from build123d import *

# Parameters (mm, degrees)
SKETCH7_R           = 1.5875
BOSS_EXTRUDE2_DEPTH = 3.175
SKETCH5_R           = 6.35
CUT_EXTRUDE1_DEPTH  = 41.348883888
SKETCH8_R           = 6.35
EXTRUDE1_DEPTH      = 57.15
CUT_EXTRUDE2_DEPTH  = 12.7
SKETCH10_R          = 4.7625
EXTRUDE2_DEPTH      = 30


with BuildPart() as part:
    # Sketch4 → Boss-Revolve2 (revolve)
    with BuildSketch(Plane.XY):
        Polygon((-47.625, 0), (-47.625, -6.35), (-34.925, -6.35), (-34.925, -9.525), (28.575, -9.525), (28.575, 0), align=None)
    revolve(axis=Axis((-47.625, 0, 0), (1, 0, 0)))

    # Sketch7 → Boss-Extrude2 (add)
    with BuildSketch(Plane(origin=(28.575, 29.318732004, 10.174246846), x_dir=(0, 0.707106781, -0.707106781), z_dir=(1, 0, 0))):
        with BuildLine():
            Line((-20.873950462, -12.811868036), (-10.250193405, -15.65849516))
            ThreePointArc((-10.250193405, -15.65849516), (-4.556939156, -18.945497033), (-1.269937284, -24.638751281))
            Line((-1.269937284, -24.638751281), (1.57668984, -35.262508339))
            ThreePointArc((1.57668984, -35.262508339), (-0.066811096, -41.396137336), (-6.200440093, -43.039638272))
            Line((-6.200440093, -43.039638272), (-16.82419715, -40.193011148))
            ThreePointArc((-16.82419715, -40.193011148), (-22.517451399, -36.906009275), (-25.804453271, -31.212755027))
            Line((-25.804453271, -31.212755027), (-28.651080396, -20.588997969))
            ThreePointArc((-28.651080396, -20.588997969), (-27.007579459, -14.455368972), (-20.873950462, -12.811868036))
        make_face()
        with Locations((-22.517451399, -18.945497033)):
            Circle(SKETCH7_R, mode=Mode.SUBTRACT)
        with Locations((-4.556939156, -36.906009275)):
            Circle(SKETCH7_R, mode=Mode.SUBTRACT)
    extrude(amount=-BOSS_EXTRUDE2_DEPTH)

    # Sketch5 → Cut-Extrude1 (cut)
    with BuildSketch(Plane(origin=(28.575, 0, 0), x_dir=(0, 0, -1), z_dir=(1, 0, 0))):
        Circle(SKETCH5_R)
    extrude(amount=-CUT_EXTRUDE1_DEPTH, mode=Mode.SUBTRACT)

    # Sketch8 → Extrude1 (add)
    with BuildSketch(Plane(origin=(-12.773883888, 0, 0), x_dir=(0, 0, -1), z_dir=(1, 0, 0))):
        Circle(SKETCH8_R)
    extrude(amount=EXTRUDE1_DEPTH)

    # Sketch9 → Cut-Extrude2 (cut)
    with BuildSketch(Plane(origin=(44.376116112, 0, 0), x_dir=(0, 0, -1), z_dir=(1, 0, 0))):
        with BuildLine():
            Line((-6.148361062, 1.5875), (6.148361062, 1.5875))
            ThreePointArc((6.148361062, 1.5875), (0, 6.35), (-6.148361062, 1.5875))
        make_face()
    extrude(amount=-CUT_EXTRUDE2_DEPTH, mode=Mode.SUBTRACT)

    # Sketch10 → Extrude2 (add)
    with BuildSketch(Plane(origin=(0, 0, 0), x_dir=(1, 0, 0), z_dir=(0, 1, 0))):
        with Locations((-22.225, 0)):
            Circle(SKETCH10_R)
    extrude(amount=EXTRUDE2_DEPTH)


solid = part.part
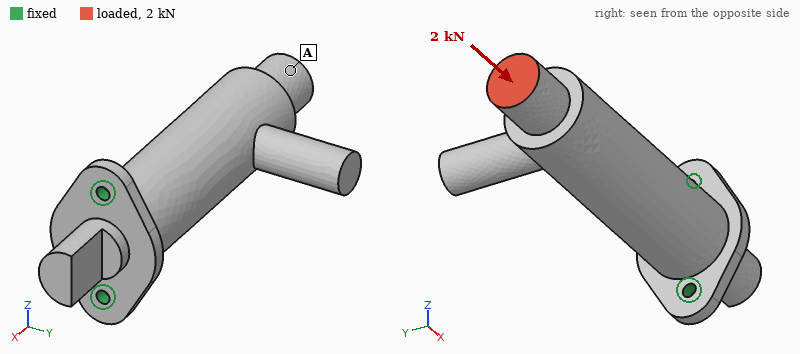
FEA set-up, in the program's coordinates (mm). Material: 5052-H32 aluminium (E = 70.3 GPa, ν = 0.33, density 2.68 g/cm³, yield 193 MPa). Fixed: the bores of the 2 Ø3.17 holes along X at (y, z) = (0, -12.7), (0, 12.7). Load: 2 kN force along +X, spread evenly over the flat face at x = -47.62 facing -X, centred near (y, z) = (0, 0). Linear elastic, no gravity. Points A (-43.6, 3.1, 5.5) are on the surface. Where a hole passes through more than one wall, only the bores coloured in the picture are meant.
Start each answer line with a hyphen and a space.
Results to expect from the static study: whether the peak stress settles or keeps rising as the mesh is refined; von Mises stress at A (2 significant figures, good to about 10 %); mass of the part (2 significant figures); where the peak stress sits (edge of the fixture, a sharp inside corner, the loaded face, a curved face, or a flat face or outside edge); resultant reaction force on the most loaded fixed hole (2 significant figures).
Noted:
- keeps rising
- 16 MPa
- 64 g
- edge of the fixture
- 1.1 kN
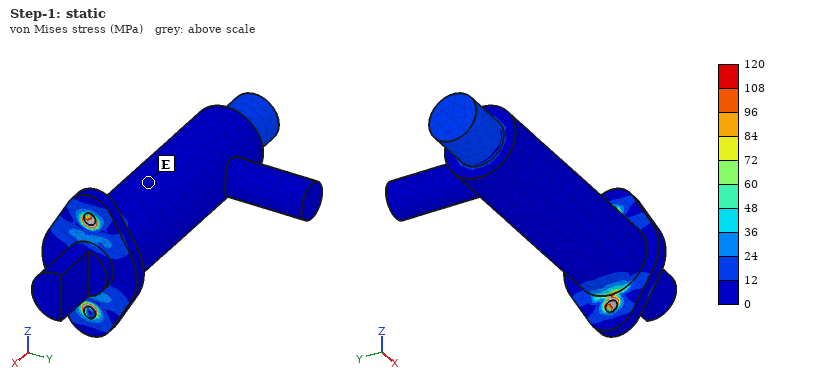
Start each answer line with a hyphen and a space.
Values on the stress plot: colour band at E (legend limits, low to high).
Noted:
- 0 to 12 MPa
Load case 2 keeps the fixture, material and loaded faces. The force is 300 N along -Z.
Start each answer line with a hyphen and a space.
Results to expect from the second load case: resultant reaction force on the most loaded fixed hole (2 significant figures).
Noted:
- 1.1 kN
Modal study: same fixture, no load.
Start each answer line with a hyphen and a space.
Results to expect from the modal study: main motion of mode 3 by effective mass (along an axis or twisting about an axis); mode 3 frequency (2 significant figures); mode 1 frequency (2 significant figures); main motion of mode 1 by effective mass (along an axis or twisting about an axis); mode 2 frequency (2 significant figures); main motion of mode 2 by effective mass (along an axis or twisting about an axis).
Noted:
- twisting about X
- 6900 Hz
- 720 Hz
- along Y
- 1900 Hz
- along Z
